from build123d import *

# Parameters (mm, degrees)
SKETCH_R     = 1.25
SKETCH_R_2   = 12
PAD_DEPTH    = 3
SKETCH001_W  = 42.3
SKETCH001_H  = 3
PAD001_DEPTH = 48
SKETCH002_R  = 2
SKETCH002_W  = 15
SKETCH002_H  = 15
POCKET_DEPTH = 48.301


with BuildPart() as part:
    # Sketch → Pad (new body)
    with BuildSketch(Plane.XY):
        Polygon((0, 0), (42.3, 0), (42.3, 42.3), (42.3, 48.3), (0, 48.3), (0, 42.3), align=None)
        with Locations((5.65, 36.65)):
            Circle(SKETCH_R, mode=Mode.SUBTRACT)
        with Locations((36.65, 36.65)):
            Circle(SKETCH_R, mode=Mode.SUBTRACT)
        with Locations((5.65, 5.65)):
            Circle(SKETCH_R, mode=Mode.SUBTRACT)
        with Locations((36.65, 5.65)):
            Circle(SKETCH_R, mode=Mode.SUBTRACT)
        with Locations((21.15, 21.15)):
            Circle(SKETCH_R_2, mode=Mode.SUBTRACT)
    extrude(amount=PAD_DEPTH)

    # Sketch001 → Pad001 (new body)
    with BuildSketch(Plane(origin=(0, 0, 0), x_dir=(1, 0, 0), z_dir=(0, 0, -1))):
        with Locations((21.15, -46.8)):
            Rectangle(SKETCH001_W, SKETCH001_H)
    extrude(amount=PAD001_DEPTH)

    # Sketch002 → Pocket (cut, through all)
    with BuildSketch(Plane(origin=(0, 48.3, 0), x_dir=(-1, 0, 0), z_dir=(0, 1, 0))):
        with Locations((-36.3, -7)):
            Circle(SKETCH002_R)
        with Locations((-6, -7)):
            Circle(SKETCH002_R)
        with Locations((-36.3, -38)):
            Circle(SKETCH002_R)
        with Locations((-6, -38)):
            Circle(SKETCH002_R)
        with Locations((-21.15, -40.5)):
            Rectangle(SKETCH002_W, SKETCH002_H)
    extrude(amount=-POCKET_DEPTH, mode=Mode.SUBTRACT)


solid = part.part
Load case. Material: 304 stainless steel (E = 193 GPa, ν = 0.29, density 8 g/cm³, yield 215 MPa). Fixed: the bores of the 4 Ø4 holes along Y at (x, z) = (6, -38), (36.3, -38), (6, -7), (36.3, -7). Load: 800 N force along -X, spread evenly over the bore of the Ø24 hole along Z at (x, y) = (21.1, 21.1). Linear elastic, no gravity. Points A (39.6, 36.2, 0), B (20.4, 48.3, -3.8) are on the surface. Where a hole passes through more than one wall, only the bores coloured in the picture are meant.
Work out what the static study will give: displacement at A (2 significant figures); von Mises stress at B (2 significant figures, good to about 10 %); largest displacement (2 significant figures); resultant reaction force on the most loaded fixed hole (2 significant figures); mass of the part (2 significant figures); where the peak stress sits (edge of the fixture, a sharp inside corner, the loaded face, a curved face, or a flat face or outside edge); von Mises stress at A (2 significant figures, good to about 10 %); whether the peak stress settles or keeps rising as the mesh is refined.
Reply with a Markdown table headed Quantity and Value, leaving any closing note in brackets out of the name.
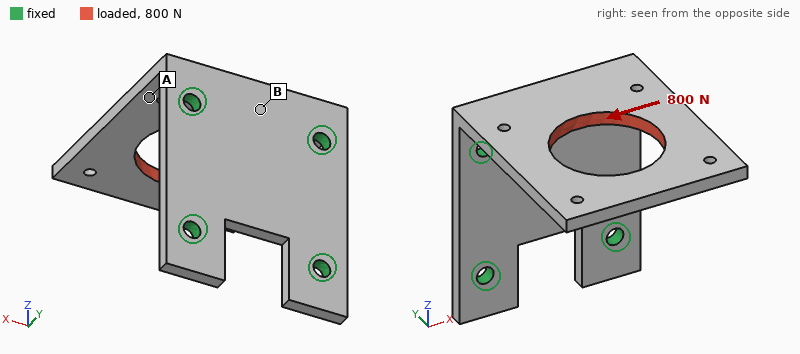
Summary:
| Quantity | Value |
|---|---|
| displacement at A | 23 µm |
| von Mises stress at B | 16 MPa |
| largest displacement | 61 µm |
| resultant reaction force on the most loaded fixed hole | 790 N |
| mass of the part | 80 g |
| where the peak stress sits | edge of the fixture |
| von Mises stress at A | 43 MPa |
| whether the peak stress settles or keeps rising as the mesh is refined | keeps rising |
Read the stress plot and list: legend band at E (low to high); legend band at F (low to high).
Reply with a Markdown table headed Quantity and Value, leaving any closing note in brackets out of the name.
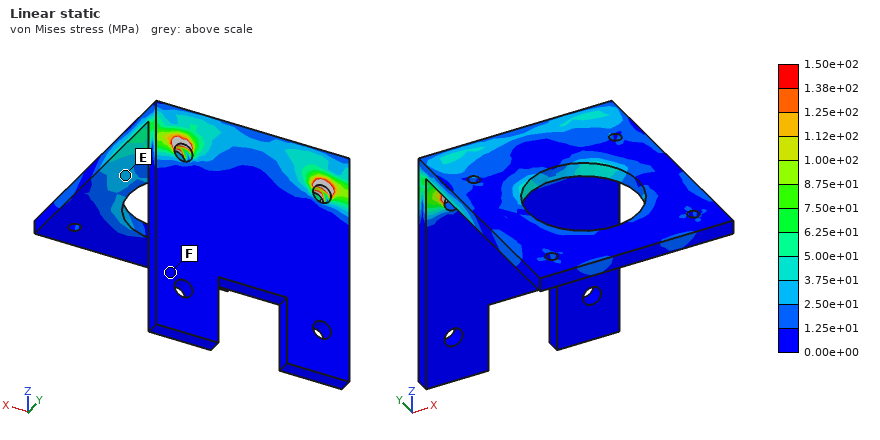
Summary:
| Quantity | Value |
|---|---|
| legend band at E | 2.50e+01 to 3.75e+01 MPa |
| legend band at F | 0.00e+00 to 1.25e+01 MPa |
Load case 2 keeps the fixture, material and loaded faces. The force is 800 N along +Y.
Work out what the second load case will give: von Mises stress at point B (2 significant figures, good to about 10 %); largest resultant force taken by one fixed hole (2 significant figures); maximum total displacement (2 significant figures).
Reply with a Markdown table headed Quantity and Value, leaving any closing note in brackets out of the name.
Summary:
| Quantity | Value |
|---|---|
| von Mises stress at point B | 25 MPa |
| largest resultant force taken by one fixed hole | 420 N |
| maximum total displacement | 73 µm |
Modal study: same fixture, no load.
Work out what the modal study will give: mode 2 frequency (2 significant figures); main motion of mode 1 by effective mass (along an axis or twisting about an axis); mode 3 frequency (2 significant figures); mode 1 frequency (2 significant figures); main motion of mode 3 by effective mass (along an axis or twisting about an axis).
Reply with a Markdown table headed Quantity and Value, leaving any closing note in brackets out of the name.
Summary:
| Quantity | Value |
|---|---|
| mode 2 frequency | 2200 Hz |
| main motion of mode 1 by effective mass | along Z |
| mode 3 frequency | 4100 Hz |
| mode 1 frequency | 870 Hz |
| main motion of mode 3 by effective mass | along X |
